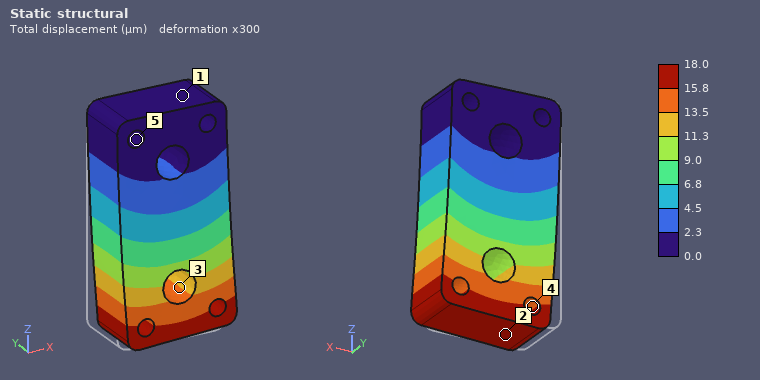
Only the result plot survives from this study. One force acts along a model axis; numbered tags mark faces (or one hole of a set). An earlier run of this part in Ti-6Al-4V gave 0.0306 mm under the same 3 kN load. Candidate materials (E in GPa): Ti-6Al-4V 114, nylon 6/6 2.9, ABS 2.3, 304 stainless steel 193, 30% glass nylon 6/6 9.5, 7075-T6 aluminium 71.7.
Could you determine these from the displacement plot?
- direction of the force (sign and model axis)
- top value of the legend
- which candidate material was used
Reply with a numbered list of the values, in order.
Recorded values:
1. +X
2. 18.0 µm
3. 304 stainless steel
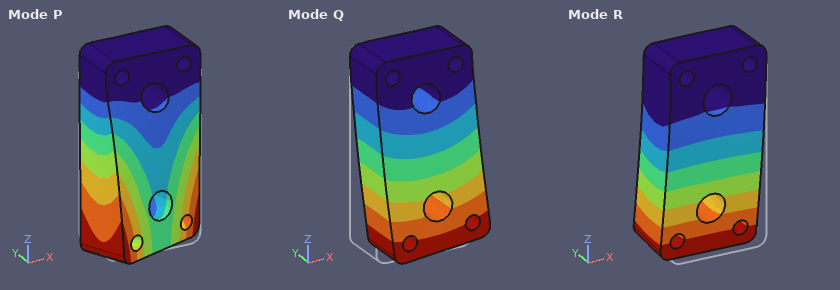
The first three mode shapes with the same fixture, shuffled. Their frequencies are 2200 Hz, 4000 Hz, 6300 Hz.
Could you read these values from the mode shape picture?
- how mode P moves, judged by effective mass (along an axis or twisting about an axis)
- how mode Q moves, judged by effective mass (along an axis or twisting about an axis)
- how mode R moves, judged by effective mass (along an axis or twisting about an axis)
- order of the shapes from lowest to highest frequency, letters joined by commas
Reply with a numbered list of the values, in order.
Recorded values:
1. twisting about Z
2. along X
3. along Y
4. R, Q, P
